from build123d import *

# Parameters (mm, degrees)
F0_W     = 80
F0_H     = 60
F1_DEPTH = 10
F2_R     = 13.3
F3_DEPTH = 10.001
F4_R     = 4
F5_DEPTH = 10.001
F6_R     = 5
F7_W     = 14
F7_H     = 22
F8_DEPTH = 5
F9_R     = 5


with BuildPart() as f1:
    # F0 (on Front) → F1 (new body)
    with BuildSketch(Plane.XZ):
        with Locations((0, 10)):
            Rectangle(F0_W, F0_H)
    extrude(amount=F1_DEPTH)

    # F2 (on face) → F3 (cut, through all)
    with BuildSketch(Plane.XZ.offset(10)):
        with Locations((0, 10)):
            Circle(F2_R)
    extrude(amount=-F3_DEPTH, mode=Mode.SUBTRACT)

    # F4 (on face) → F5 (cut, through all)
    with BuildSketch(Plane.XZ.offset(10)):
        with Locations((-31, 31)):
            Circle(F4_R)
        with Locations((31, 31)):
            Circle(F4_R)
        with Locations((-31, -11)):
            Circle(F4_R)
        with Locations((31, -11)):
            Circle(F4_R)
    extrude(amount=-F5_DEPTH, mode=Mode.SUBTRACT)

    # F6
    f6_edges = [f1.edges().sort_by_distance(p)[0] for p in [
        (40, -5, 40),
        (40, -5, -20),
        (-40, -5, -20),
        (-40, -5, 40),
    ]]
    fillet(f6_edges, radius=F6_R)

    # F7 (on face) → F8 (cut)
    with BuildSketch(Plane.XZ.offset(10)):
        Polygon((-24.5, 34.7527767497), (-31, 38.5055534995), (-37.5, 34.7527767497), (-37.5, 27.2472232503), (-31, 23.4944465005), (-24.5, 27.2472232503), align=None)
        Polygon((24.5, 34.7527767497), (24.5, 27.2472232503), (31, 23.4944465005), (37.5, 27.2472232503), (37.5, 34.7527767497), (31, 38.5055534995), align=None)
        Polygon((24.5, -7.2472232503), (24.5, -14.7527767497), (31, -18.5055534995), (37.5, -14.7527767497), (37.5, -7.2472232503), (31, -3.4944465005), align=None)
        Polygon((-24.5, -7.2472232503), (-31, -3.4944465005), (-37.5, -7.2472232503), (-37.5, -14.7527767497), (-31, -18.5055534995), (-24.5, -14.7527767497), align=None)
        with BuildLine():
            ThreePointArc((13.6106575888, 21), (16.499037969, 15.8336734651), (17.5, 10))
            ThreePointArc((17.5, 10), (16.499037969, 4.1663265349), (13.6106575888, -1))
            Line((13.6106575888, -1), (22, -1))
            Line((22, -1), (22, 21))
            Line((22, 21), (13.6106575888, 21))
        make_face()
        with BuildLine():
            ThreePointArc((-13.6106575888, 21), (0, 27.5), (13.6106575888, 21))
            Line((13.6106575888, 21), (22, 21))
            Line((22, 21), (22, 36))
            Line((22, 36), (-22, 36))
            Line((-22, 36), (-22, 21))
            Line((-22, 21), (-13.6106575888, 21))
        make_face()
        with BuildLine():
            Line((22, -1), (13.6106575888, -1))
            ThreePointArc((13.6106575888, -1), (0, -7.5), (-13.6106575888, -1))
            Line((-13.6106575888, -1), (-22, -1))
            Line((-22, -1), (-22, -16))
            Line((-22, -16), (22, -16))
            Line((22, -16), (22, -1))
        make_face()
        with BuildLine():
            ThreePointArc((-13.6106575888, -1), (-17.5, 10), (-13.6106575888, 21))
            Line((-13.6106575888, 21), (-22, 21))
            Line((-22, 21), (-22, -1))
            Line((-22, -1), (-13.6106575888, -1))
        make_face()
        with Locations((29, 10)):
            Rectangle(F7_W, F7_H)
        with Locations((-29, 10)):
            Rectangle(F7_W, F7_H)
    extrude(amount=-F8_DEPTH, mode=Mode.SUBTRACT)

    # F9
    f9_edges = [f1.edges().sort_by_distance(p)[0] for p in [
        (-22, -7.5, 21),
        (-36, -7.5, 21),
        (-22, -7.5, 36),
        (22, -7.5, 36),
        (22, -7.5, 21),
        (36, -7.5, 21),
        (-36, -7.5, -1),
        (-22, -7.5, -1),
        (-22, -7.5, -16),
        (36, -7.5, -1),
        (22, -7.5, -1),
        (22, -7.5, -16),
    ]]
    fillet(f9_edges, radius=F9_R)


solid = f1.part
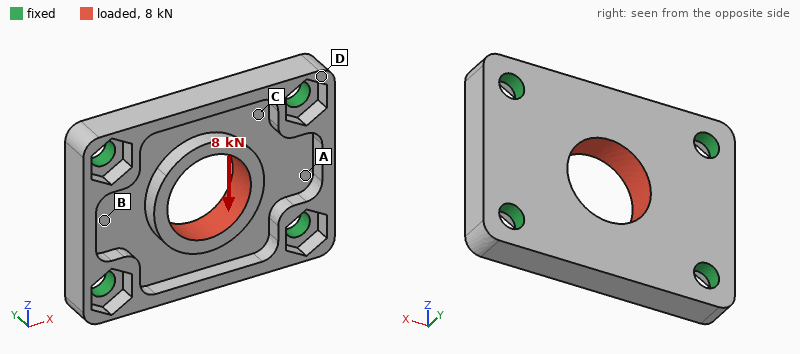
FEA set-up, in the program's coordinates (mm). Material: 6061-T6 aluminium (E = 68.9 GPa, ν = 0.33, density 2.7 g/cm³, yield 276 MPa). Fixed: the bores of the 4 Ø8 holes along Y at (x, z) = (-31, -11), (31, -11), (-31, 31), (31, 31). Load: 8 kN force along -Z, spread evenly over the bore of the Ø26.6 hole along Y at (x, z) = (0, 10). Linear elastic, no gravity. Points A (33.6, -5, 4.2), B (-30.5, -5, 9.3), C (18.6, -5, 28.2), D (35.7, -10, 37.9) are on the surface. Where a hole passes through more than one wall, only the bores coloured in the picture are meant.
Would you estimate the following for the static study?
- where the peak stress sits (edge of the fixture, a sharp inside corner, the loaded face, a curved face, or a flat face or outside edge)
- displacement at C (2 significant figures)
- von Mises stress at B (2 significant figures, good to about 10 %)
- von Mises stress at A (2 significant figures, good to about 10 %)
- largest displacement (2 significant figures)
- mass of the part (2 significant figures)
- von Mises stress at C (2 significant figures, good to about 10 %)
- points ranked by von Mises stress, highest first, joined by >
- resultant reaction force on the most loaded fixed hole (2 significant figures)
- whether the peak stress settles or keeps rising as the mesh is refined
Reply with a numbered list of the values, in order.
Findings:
1. edge of the fixture
2. 8.2 µm
3. 18 MPa
4. 12 MPa
5. 26 µm
6. 77 g
7. 27 MPa
8. C > B > A > D
9. 2.3 kN
10. keeps rising
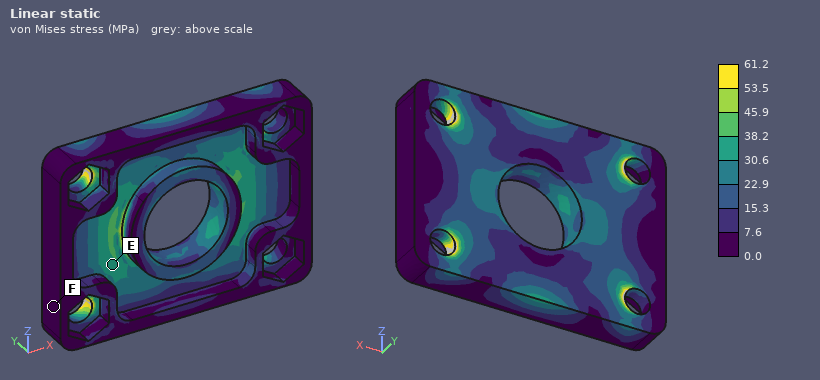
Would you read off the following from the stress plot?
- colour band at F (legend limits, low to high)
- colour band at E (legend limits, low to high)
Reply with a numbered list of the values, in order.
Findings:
1. 0.0 to 7.6 MPa
2. 30.6 to 38.2 MPa
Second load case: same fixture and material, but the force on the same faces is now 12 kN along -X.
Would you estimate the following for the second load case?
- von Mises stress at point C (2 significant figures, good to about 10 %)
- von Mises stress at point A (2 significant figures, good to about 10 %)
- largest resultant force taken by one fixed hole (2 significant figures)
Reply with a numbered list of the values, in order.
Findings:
1. 33 MPa
2. 7.5 MPa
3. 3.1 kN
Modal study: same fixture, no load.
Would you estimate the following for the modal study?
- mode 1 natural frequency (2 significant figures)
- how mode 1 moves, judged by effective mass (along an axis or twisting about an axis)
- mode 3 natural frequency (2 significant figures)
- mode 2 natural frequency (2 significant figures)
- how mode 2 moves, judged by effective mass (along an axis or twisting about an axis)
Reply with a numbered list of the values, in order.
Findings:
1. 9000 Hz
2. along Y
3. 14 kHz
4. 10 kHz
5. twisting about X
